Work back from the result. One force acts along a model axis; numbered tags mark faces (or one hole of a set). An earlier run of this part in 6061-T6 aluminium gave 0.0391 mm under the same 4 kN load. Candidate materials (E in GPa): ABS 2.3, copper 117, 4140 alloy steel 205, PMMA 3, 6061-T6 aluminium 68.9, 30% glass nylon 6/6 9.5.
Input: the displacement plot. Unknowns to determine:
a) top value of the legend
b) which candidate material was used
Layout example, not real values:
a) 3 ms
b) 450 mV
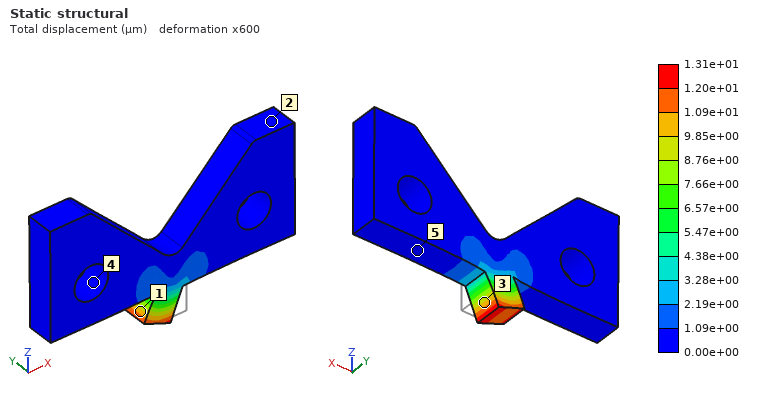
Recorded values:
a) 1.31e+01 µm
b) 4140 alloy steel
